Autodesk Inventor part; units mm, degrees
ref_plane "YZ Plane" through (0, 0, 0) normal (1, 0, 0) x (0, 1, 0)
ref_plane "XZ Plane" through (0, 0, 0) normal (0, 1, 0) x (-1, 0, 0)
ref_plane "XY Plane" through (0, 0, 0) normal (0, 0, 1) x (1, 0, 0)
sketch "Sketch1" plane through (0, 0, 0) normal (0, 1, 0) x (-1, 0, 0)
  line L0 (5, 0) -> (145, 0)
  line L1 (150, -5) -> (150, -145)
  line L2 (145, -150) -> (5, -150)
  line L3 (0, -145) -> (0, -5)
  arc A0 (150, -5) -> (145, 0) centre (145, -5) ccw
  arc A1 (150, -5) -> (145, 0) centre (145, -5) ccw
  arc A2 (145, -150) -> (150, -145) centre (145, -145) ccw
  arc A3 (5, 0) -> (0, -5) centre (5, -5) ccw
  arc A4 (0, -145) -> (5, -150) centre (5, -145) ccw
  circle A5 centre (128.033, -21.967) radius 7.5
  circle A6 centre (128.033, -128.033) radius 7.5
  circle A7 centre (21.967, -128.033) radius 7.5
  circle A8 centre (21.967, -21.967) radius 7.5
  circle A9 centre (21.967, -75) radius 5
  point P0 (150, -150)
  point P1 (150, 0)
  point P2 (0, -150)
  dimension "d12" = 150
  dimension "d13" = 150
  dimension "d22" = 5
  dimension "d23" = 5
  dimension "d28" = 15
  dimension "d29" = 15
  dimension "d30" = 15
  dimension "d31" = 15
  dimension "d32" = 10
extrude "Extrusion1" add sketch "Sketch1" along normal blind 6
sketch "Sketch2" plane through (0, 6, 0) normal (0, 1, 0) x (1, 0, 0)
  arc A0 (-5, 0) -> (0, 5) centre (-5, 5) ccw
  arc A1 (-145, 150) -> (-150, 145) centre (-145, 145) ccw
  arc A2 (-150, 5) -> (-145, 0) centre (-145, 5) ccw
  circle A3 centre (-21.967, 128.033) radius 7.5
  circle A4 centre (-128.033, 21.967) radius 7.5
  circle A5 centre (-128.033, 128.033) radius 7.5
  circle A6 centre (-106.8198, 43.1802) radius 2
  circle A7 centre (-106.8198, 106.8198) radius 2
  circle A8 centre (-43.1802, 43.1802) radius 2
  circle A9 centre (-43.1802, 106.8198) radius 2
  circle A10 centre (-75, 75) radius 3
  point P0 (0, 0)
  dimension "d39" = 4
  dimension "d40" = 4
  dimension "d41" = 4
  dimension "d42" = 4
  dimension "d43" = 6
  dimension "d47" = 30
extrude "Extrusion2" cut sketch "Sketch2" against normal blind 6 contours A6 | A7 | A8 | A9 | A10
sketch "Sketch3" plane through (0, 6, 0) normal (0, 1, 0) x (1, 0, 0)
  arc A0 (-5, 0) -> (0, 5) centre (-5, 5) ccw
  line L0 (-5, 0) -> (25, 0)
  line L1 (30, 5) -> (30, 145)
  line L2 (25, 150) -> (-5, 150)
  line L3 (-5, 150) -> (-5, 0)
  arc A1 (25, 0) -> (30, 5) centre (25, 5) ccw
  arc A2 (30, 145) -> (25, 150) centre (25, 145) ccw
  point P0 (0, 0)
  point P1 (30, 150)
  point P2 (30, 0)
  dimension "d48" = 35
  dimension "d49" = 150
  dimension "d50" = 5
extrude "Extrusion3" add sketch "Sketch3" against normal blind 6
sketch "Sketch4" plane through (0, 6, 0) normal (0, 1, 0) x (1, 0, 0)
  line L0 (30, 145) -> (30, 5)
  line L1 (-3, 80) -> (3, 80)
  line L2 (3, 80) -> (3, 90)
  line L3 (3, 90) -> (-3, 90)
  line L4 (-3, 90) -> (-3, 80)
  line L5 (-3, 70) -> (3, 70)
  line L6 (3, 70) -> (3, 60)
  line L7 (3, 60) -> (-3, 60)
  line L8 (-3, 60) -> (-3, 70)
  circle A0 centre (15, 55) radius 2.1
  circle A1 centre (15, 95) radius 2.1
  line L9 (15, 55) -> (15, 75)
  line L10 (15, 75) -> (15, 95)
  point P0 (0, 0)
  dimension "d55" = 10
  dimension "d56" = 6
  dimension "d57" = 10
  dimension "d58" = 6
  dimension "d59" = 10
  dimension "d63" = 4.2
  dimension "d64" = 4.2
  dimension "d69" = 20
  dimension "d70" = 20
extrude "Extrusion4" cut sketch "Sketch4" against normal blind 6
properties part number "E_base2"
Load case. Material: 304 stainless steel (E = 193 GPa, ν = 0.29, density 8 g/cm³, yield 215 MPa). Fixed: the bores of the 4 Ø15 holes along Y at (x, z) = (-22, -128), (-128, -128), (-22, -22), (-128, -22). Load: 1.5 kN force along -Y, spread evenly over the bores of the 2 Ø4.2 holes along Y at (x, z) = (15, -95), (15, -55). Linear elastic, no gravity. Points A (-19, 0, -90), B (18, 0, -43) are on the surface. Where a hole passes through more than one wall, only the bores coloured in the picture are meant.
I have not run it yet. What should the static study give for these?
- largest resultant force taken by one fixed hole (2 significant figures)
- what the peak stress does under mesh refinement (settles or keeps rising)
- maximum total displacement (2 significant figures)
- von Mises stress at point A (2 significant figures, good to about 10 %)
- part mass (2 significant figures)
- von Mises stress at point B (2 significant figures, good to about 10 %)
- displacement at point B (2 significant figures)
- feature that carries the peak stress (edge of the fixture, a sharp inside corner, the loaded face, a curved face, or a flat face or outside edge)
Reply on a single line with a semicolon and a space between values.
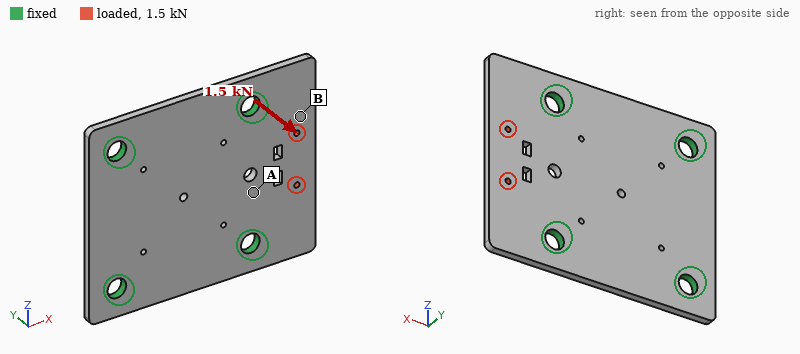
800 N; keeps rising; 0.14 mm; 36 MPa; 1.2 kg; 14 MPa; 0.078 mm; edge of the fixture
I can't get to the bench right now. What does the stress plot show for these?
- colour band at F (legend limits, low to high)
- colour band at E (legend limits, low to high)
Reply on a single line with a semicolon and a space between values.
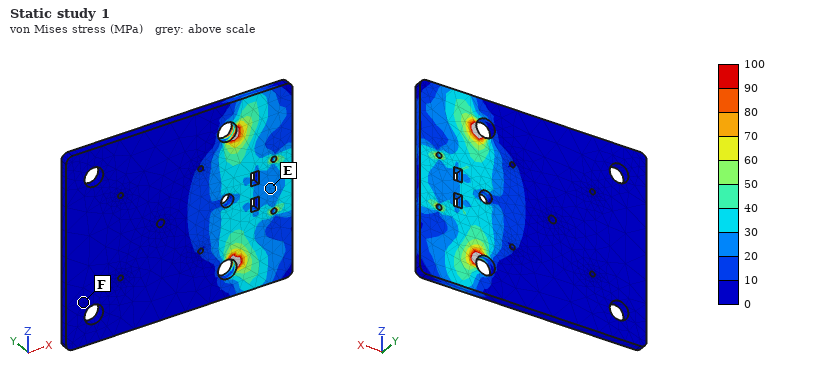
0 to 10 MPa; 20 to 30 MPa
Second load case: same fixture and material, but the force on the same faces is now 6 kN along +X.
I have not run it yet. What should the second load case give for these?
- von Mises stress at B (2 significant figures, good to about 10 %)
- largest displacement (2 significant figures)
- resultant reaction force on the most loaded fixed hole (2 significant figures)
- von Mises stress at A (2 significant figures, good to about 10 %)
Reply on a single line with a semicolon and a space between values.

10 MPa; 5.5 µm; 2.5 kN; 7.1 MPa
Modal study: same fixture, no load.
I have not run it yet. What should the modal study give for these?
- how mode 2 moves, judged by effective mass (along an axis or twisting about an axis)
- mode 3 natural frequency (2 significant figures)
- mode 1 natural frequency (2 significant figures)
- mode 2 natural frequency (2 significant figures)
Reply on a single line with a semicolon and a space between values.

along Y; 2500 Hz; 1700 Hz; 2200 Hz
